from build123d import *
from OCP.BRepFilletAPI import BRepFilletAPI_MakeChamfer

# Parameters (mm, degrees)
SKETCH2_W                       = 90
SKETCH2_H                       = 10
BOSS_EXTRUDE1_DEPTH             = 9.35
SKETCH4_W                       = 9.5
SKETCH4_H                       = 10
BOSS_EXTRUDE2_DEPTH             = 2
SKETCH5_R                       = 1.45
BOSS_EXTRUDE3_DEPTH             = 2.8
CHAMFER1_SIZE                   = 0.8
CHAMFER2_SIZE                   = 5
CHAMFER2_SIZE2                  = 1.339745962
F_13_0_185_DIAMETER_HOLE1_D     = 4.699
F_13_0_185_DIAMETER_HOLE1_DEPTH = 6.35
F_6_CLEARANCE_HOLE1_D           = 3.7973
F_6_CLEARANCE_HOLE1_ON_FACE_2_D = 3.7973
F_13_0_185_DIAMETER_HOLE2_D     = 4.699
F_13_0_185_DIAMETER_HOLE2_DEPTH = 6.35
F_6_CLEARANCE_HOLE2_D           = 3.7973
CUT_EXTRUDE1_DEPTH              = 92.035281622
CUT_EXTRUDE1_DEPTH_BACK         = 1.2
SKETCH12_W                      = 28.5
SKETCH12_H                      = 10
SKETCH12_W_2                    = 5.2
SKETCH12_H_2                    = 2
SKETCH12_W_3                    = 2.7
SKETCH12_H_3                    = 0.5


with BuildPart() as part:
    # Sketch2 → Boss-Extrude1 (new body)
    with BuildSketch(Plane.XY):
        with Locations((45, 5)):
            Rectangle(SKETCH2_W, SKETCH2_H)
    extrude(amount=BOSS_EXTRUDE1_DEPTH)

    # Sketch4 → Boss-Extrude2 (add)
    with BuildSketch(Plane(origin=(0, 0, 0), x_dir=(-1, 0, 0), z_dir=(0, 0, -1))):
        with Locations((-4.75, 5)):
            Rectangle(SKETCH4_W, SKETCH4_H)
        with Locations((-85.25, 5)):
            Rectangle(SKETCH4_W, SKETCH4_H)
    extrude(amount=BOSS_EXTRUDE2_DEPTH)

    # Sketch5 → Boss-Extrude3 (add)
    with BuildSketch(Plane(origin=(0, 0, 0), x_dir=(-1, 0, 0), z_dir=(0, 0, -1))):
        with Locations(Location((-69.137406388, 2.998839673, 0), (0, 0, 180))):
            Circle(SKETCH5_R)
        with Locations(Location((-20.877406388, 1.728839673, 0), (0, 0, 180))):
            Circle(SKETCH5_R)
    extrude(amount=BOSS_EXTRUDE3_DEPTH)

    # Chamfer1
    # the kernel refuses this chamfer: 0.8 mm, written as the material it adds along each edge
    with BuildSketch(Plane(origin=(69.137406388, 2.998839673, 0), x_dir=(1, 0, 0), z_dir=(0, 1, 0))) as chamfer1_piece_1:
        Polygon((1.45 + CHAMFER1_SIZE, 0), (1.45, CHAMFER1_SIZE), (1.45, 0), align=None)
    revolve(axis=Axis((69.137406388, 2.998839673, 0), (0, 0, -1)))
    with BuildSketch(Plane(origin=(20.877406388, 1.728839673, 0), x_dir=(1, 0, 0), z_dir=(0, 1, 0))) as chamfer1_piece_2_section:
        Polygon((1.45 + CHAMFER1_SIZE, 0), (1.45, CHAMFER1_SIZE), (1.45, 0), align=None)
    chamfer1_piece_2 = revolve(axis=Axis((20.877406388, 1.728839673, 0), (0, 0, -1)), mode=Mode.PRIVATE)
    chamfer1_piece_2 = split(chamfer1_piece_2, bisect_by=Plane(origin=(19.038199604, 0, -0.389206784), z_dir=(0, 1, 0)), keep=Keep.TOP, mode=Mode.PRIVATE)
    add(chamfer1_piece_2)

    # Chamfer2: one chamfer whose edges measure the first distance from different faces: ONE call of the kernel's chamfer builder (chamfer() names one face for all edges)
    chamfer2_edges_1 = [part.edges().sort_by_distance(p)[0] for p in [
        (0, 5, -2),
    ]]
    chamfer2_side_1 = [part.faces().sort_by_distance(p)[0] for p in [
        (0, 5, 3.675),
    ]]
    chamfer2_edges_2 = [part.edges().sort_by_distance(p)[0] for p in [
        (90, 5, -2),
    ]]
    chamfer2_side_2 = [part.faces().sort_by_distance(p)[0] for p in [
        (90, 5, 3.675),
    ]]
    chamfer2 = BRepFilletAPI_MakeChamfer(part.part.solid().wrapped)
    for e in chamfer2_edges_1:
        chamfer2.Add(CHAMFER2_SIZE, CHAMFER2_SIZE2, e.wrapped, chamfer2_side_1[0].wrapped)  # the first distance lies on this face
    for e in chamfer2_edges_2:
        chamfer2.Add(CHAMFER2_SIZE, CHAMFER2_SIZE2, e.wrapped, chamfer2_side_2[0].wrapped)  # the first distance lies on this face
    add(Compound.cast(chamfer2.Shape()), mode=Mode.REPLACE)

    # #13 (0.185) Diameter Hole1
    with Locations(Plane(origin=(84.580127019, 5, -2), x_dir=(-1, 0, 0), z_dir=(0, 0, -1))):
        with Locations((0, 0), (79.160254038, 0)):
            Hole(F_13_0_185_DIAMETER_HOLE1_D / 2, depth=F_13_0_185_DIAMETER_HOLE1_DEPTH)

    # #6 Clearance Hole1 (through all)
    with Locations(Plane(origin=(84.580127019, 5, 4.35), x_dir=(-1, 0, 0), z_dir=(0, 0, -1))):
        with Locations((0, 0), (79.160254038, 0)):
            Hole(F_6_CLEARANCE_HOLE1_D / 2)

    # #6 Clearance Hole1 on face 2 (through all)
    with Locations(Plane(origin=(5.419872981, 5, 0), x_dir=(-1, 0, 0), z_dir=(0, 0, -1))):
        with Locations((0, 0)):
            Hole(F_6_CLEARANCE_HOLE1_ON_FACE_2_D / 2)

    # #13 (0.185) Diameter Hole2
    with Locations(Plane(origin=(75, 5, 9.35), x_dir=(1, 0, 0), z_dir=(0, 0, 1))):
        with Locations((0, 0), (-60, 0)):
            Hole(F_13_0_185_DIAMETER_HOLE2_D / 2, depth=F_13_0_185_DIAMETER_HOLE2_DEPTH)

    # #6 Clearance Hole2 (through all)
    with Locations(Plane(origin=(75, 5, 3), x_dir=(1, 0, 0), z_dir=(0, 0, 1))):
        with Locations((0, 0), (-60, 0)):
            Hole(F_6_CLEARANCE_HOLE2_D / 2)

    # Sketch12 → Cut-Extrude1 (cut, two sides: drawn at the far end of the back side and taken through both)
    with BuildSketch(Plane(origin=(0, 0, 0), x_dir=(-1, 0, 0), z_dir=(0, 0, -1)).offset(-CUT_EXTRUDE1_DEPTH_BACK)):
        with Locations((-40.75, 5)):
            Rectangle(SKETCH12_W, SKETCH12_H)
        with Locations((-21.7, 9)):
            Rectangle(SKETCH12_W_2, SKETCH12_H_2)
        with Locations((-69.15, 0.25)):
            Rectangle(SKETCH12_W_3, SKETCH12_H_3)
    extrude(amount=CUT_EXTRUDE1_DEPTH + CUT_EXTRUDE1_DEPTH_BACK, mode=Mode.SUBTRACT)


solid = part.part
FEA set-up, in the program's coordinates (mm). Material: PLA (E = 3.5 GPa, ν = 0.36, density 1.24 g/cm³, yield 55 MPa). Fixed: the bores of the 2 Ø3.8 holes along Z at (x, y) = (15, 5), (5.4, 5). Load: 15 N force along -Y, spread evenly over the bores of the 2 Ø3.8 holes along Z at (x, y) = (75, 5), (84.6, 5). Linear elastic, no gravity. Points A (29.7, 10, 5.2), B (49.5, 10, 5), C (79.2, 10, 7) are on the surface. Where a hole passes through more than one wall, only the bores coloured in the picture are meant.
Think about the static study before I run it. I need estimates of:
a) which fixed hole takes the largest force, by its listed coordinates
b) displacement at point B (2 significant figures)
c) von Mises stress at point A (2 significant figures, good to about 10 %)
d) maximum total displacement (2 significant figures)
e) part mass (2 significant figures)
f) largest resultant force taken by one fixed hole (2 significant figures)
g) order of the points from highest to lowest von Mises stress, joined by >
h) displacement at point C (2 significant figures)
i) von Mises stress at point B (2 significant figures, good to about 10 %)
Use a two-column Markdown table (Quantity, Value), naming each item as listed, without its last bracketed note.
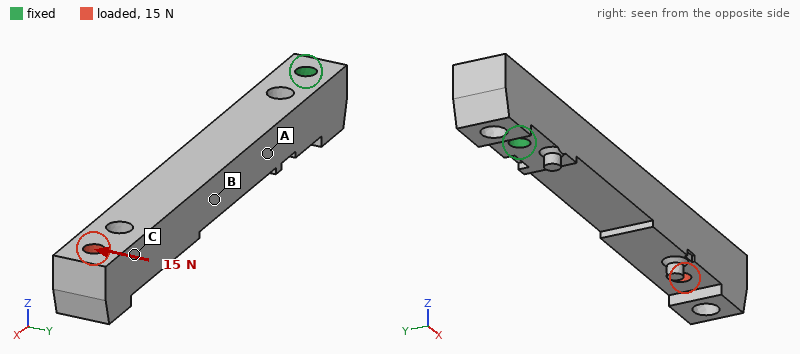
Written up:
| Quantity | Value |
|---|---|
| which fixed hole takes the largest force, by its listed coordinates | (15, 5) |
| displacement at point B | 0.27 mm |
| von Mises stress at point A | 5.6 MPa |
| maximum total displacement | 0.86 mm |
| part mass | 9.7 g |
| largest resultant force taken by one fixed hole | 61 N |
| order of the points from highest to lowest von Mises stress, joined by > | A > B > C |
| displacement at point C | 0.69 mm |
| von Mises stress at point B | 3.5 MPa |
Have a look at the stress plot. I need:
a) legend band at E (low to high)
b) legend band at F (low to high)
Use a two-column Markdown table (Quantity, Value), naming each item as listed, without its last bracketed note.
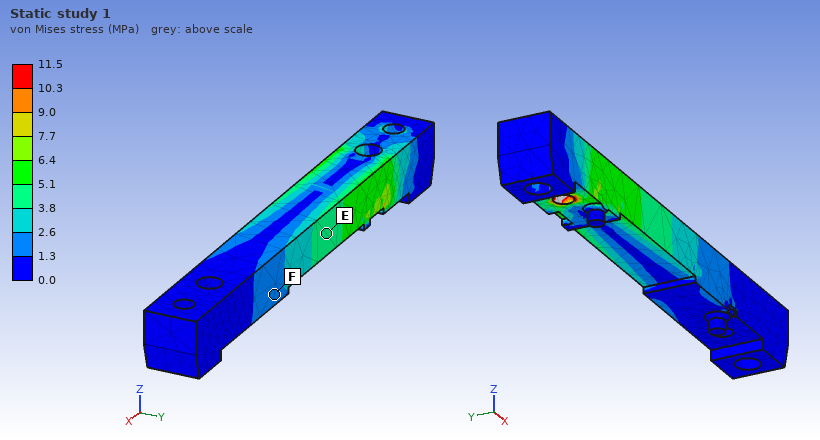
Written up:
| Quantity | Value |
|---|---|
| legend band at E | 3.8 to 5.1 MPa |
| legend band at F | 1.3 to 2.6 MPa |
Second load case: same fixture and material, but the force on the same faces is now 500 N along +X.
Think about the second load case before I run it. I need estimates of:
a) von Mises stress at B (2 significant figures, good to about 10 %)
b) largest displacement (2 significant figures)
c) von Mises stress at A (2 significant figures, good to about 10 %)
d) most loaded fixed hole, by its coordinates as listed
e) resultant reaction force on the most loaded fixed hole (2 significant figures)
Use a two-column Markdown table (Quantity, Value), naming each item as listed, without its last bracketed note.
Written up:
| Quantity | Value |
|---|---|
| von Mises stress at B | 6.2 MPa |
| largest displacement | 0.20 mm |
| von Mises stress at A | 5.9 MPa |
| most loaded fixed hole, by its coordinates as listed | (15, 5) |
| resultant reaction force on the most loaded fixed hole | 280 N |
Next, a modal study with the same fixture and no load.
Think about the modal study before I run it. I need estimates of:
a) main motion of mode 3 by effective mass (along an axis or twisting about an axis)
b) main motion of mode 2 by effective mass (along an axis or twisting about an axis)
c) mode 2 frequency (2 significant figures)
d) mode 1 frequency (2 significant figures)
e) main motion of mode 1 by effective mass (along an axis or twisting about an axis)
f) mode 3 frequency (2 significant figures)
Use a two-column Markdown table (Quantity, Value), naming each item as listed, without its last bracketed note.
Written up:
| Quantity | Value |
|---|---|
| main motion of mode 3 by effective mass | along Z |
| main motion of mode 2 by effective mass | along Y |
| mode 2 frequency | 420 Hz |
| mode 1 frequency | 370 Hz |
| main motion of mode 1 by effective mass | along Z |
| mode 3 frequency | 2300 Hz |
